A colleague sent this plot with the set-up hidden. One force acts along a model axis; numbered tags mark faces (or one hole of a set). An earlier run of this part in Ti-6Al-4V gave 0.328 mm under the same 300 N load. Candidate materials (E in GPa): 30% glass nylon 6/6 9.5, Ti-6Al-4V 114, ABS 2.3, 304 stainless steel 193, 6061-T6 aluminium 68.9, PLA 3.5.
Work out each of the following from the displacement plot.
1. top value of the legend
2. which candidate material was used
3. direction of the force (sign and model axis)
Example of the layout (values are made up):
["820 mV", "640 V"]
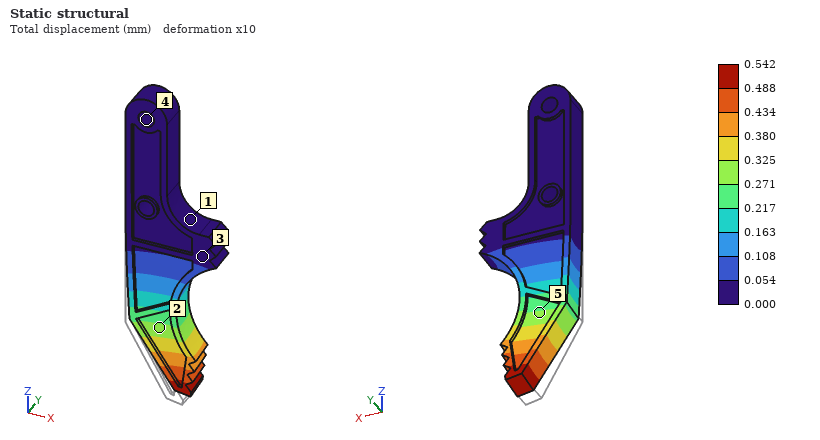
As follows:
["0.542 mm", "6061-T6 aluminium", "+Y"]
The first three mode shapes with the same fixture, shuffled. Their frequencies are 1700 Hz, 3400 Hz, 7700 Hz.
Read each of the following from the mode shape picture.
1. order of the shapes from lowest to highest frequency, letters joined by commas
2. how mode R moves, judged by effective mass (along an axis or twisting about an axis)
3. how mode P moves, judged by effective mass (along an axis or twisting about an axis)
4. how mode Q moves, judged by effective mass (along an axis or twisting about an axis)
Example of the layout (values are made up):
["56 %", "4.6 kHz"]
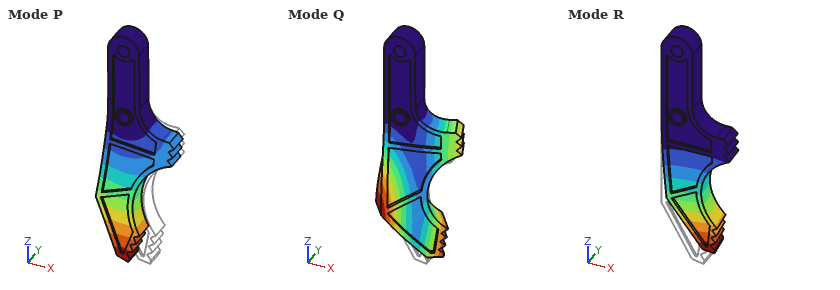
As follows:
["R, P, Q", "along Y", "along X", "twisting about Z"]
